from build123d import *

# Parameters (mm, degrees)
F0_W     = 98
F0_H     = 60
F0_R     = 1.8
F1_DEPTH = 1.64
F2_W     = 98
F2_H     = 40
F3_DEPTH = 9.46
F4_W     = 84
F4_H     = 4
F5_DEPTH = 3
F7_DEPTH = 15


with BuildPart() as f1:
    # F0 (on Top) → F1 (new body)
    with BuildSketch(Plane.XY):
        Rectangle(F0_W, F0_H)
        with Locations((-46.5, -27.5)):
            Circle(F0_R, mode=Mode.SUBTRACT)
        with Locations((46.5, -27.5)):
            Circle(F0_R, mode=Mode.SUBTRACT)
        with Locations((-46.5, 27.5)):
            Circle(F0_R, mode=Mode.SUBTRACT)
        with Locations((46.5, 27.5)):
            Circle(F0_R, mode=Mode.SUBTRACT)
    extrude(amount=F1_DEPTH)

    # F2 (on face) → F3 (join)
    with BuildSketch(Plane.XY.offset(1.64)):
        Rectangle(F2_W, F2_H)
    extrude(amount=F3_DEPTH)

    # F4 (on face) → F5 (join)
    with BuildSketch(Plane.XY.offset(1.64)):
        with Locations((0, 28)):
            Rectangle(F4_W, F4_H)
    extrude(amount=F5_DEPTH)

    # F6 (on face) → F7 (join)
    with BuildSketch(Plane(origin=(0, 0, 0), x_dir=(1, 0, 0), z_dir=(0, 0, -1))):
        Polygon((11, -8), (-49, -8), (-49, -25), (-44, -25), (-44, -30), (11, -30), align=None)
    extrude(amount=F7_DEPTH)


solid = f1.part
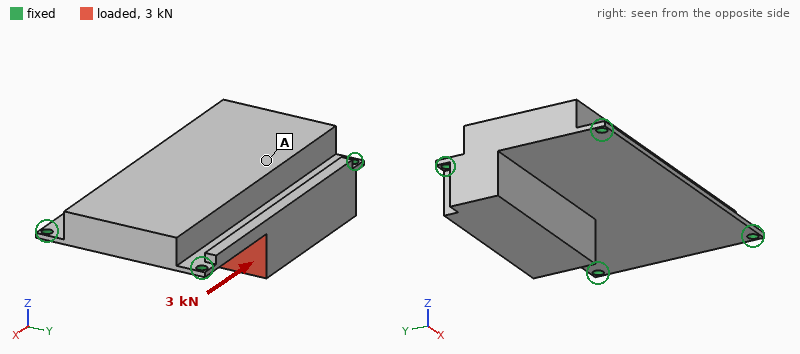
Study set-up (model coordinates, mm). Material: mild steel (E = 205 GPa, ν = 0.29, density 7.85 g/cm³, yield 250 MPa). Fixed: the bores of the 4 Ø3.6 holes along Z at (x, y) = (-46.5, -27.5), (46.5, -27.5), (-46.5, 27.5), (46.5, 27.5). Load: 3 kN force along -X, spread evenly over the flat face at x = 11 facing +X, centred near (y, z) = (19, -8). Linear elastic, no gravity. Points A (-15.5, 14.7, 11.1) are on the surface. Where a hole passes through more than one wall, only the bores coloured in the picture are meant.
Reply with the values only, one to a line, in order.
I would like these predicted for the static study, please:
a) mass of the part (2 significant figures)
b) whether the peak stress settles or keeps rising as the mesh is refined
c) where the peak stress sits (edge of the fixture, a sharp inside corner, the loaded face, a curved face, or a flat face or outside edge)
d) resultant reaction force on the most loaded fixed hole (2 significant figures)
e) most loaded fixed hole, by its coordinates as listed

530 g
keeps rising
edge of the fixture
1.6 kN
(-46.5, 27.5)
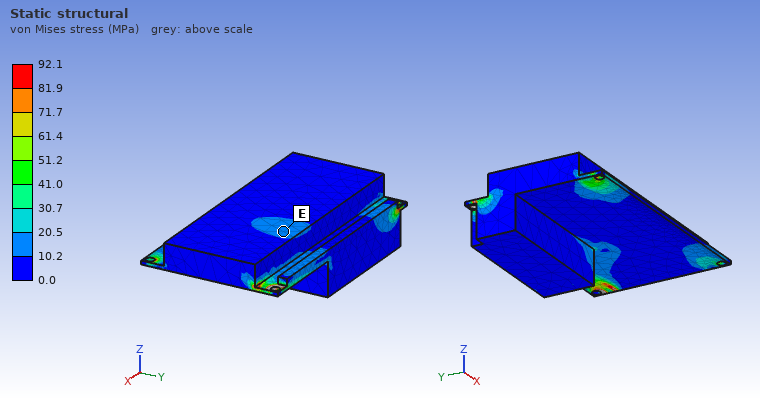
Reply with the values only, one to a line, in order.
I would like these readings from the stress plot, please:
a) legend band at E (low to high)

10.2 to 20.5 MPa
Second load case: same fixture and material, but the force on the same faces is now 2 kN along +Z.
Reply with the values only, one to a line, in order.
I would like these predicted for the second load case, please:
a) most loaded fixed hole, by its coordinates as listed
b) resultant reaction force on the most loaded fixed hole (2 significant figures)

(46.5, 27.5)
1.1 kN
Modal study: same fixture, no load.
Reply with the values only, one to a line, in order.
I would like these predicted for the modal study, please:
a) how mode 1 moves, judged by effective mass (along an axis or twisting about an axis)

along Z
